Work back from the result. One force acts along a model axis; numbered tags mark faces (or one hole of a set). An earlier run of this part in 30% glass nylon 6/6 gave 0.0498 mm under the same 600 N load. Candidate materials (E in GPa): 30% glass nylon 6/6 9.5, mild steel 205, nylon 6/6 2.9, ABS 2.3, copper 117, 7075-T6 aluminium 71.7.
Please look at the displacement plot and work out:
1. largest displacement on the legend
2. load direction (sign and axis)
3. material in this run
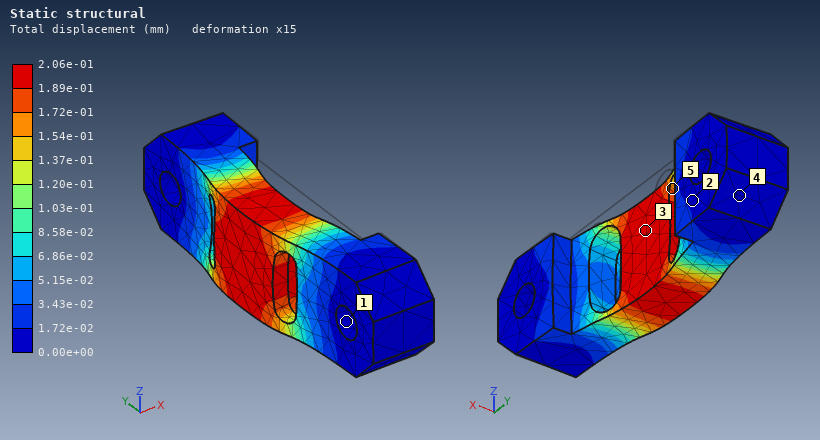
2.06e-01 mm
-X
ABS
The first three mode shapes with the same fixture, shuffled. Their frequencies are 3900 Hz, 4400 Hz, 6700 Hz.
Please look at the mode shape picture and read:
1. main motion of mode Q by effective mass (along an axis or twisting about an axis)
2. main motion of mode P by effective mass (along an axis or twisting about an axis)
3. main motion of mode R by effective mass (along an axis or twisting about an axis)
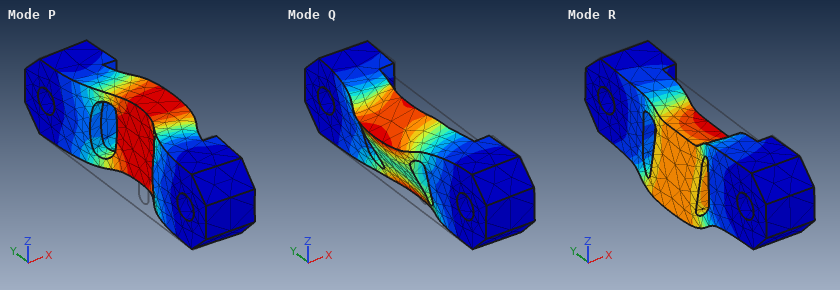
twisting about Y
along X
along Z
